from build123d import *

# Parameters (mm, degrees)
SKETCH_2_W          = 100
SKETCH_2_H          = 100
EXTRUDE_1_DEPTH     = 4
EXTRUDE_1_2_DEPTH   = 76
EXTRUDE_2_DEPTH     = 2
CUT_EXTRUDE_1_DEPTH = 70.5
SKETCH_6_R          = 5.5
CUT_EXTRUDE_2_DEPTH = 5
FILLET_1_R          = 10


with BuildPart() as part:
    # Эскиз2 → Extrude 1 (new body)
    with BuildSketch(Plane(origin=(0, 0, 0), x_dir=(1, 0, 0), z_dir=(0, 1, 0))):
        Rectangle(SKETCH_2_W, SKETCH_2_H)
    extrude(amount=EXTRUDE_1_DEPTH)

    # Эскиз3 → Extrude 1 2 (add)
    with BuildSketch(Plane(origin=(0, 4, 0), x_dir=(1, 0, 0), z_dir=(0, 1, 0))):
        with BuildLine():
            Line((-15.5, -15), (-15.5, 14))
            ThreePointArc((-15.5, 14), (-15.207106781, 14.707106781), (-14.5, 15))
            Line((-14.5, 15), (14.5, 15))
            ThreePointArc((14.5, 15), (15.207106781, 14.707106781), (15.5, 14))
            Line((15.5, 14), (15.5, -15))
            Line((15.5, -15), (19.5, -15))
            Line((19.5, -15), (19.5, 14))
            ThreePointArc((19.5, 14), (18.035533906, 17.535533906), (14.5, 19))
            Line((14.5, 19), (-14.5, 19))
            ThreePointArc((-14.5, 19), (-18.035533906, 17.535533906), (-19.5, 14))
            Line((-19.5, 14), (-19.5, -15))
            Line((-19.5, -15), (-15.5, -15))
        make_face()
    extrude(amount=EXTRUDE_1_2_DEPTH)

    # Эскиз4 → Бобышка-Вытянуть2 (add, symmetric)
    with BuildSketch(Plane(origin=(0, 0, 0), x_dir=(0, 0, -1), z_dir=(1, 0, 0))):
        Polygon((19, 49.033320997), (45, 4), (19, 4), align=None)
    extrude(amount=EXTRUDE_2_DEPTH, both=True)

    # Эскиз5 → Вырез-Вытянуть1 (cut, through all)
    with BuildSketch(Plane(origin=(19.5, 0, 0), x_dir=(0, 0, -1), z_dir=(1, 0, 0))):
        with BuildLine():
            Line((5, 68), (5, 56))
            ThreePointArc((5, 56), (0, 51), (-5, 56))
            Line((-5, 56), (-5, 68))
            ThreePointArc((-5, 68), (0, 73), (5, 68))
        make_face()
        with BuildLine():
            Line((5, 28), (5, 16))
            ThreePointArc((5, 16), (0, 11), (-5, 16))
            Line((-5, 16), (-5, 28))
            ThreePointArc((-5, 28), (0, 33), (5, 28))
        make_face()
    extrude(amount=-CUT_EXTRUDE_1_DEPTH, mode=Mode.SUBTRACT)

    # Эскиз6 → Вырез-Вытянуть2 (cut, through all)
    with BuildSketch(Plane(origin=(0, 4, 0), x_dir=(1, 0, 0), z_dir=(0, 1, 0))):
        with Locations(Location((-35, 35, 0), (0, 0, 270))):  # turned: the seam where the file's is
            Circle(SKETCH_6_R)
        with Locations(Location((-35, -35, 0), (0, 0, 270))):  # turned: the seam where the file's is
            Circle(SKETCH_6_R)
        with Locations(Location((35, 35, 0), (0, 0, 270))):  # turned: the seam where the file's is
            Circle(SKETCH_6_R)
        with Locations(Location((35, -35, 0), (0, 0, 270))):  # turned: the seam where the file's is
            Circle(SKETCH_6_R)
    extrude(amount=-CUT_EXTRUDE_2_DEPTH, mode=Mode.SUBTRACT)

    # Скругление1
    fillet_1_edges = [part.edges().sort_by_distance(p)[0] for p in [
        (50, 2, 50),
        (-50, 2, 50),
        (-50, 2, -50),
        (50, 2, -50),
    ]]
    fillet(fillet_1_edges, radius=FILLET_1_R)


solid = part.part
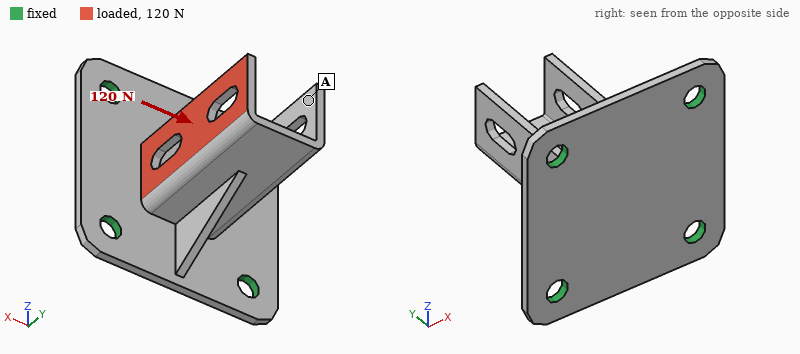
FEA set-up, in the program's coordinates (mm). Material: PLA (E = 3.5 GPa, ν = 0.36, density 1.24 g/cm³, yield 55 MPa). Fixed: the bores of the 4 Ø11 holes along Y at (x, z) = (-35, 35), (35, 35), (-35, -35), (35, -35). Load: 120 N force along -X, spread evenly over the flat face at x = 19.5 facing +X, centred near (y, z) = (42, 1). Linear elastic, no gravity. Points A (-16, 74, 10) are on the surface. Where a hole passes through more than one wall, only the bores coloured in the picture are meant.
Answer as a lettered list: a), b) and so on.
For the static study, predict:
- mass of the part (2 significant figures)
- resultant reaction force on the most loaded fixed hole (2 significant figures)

a) 83 g
b) 83 N
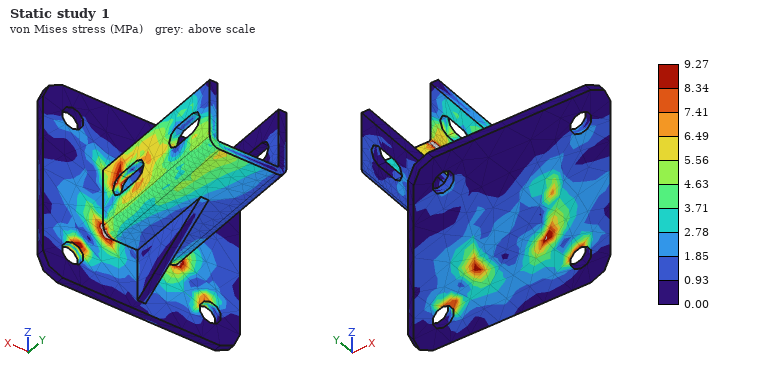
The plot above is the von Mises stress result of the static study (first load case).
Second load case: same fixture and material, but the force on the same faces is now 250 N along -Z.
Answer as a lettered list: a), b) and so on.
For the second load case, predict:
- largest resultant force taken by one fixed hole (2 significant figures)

a) 150 N
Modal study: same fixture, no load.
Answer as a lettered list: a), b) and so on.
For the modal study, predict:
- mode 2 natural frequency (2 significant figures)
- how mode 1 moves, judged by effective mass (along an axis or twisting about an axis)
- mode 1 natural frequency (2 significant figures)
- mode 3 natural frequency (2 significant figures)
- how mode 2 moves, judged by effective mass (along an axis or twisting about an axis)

a) 590 Hz
b) along X
c) 420 Hz
d) 810 Hz
e) along Z
